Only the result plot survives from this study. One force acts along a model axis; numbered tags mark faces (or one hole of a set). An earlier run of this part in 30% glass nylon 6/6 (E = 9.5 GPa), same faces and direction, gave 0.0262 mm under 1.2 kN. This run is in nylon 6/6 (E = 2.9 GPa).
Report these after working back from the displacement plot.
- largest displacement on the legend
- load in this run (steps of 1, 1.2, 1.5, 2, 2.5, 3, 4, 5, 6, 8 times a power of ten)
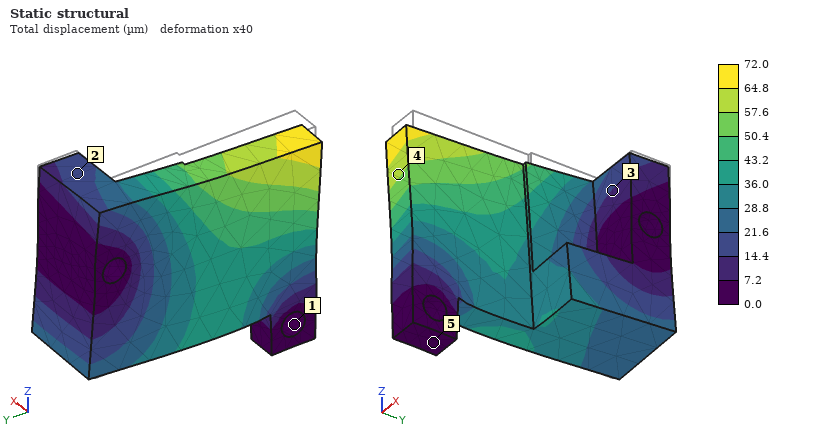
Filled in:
72.0 µm
1 kN
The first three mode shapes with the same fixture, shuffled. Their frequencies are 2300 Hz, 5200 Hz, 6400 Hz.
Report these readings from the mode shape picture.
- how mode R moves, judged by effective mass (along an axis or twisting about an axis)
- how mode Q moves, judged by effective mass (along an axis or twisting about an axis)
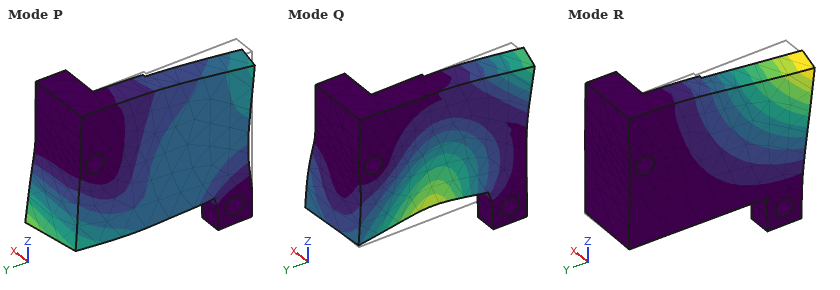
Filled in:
along X
along X
